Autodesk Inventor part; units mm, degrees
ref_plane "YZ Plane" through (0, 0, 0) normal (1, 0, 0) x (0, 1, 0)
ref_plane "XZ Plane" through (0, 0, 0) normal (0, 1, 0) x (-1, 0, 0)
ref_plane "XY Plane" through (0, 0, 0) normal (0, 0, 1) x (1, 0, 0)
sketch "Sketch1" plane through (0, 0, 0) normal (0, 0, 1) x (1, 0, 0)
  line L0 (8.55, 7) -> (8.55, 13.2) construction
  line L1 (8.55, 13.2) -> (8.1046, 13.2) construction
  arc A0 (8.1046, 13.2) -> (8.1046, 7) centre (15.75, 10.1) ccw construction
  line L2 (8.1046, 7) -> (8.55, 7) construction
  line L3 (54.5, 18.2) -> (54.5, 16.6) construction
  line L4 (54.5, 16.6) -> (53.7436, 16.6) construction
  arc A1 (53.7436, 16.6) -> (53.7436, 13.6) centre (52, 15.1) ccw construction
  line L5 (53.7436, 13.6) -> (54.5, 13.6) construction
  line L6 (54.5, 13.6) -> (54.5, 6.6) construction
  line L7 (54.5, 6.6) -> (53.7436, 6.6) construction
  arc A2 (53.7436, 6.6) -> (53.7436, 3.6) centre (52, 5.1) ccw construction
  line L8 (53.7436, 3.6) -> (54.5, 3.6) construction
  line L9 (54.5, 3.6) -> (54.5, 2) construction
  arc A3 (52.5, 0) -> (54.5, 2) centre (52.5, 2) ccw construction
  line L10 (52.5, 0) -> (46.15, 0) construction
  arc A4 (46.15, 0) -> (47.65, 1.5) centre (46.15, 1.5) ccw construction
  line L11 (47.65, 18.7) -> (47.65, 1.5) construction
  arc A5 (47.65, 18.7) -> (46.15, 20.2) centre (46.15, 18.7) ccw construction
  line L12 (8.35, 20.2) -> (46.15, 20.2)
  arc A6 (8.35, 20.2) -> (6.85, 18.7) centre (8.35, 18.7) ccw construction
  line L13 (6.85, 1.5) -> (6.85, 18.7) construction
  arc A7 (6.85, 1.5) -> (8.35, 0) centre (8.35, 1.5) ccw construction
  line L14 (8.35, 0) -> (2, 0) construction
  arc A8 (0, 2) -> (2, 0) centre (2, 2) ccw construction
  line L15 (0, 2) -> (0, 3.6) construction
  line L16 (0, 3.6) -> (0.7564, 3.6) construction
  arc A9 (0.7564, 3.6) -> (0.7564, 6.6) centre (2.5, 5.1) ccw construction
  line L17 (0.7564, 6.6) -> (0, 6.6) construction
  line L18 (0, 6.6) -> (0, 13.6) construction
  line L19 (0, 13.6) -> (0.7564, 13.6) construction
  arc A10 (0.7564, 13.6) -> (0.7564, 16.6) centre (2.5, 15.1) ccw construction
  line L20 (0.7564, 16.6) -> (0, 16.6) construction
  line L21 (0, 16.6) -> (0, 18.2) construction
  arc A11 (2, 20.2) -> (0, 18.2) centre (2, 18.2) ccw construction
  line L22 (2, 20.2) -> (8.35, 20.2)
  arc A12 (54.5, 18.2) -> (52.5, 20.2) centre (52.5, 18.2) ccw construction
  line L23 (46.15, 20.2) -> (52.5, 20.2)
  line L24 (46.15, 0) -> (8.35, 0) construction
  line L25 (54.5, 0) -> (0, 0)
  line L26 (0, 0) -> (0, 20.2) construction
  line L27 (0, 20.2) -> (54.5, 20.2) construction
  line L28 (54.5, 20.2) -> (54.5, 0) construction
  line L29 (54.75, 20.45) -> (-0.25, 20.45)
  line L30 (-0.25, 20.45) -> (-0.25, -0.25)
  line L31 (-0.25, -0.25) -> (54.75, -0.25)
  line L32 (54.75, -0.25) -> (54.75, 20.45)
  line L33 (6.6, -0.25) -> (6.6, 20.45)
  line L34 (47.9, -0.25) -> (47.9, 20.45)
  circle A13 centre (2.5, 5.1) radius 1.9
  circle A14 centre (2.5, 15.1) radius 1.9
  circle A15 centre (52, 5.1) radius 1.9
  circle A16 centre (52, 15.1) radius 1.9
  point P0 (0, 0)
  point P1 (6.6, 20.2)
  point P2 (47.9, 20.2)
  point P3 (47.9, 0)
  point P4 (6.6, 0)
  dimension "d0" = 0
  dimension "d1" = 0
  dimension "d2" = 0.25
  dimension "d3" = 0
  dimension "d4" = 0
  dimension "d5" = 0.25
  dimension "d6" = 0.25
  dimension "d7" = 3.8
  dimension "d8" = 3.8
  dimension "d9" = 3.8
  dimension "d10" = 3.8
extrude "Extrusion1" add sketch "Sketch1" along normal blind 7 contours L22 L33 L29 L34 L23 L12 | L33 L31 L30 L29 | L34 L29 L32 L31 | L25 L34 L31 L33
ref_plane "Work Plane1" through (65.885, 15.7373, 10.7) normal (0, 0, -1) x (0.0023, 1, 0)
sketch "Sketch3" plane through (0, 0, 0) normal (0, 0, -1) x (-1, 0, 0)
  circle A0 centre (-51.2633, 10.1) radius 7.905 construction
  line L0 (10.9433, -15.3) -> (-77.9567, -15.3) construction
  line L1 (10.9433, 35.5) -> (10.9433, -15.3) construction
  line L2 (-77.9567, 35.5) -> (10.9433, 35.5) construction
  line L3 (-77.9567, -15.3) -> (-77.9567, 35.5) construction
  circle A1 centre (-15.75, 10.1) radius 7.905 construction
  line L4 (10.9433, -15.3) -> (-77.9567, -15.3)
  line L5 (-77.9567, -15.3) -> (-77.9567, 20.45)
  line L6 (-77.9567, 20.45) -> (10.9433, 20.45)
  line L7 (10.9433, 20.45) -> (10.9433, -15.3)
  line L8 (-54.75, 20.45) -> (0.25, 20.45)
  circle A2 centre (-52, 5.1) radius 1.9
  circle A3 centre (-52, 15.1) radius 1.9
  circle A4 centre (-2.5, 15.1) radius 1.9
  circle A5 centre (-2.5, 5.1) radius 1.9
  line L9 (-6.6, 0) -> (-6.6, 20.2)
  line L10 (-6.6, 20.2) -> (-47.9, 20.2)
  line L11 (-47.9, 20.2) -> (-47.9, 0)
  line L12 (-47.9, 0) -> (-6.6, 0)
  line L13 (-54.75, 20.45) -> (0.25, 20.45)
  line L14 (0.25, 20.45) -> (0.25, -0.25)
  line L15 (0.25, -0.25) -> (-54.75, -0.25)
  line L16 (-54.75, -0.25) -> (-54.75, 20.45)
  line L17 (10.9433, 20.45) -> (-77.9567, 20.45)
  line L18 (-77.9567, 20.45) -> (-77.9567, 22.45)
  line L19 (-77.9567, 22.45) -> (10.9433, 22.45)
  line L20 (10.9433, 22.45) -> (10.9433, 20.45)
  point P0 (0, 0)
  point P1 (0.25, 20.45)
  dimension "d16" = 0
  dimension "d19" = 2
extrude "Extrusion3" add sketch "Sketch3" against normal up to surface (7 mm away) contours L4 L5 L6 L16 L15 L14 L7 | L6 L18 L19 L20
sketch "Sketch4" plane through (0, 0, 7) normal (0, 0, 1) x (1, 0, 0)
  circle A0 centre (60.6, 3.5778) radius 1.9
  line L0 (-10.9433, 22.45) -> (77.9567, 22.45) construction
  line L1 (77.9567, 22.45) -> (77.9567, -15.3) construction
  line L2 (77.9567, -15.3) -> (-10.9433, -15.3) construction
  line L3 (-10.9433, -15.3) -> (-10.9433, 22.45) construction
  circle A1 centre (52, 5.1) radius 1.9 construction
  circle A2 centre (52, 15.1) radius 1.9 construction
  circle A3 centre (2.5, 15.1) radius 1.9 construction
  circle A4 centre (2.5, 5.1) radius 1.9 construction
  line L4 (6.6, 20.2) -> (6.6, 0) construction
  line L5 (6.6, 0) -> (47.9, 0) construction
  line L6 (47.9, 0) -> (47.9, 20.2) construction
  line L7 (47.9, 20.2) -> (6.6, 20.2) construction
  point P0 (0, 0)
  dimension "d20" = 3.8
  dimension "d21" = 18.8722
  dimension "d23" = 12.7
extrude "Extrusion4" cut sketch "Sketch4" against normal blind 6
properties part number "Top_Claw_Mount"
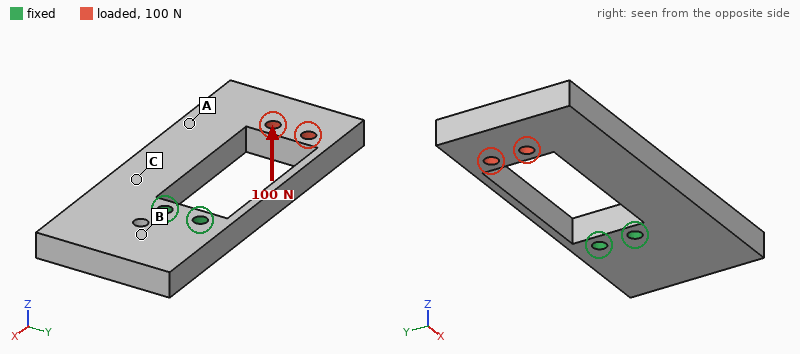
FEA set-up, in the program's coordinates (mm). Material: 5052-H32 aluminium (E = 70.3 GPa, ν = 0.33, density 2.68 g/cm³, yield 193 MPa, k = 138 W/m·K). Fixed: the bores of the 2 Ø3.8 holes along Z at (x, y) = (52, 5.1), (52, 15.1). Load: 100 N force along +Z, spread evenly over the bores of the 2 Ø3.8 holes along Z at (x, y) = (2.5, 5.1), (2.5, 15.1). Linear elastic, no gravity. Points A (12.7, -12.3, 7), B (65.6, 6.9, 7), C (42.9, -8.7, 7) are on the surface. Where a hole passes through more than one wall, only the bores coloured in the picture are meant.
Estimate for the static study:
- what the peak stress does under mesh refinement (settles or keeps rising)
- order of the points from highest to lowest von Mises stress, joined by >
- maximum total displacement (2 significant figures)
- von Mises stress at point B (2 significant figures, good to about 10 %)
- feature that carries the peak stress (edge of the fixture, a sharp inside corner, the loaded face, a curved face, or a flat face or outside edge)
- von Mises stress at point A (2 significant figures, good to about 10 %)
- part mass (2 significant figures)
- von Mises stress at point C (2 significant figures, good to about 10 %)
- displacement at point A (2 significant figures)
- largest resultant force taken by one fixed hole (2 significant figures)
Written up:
keeps rising
C > A > B
0.25 mm
5.1 MPa
edge of the fixture
10.0 MPa
46 g
24 MPa
0.11 mm
50 N
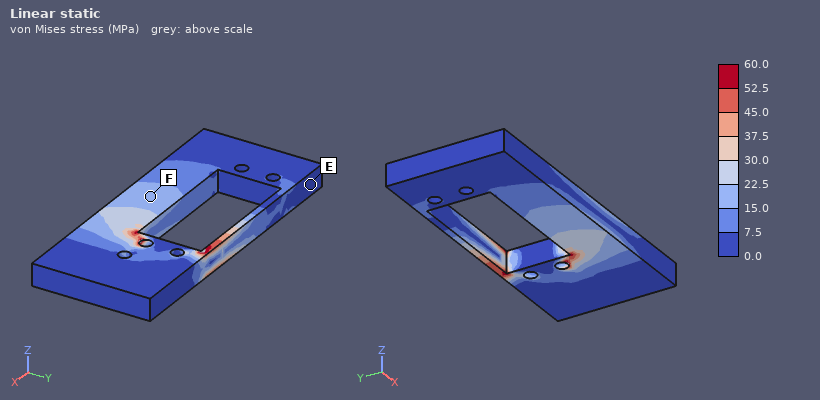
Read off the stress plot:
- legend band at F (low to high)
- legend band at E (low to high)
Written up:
15.0 to 22.5 MPa
0.0 to 7.5 MPa
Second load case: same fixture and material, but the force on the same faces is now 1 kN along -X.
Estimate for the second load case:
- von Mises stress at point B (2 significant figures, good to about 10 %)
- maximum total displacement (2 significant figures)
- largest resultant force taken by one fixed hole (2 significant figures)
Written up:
2.9 MPa
37 µm
530 N
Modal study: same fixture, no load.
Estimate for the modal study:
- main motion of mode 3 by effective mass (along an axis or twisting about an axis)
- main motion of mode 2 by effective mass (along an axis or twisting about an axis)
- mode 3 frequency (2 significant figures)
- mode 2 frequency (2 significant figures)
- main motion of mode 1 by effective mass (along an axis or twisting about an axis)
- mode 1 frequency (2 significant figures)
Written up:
twisting about X
along Y
2900 Hz
2300 Hz
along Z
910 Hz
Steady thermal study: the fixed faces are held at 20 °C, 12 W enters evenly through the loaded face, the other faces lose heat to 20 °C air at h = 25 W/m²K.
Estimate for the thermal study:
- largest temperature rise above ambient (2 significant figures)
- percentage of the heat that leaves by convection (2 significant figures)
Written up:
40 K
25 %
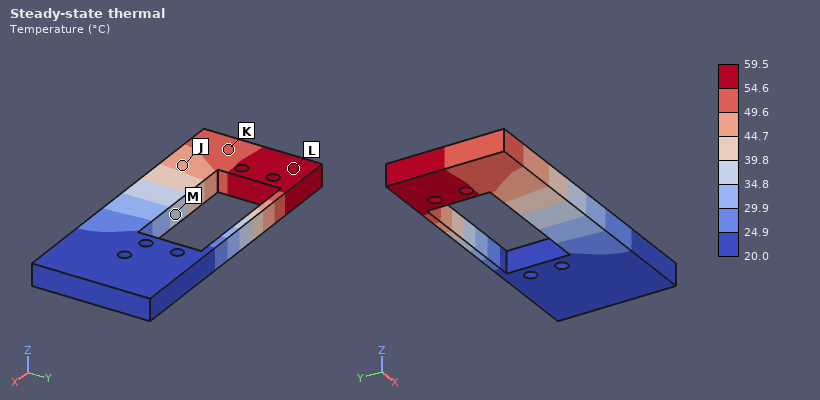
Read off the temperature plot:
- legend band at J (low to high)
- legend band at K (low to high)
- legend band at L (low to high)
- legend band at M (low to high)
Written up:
44.7 to 49.6 °C
49.6 to 54.6 °C
54.6 to 59.5 °C
34.8 to 39.8 °C
